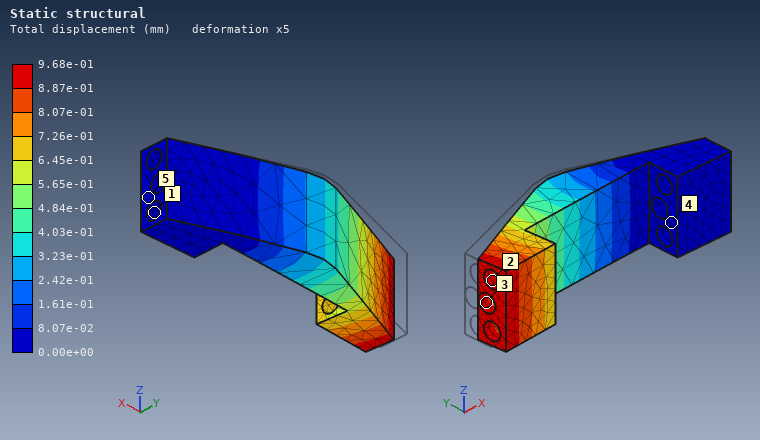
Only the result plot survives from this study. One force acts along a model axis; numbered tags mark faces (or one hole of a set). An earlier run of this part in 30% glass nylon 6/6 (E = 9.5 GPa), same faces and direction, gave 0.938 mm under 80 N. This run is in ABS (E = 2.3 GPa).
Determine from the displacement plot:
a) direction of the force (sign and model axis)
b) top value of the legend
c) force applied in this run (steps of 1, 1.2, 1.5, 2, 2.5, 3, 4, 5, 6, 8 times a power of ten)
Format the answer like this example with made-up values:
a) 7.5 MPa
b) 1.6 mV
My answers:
a) -Y
b) 9.68e-01 mm
c) 20 N
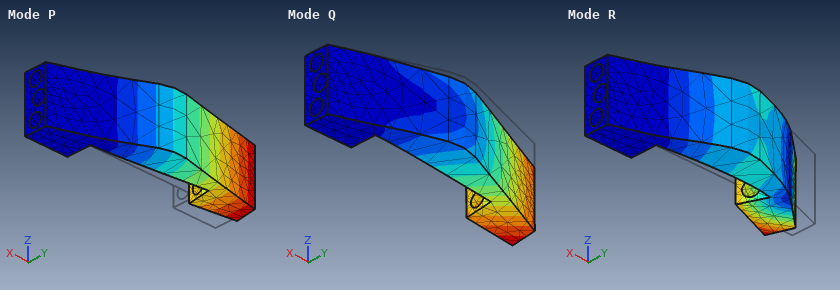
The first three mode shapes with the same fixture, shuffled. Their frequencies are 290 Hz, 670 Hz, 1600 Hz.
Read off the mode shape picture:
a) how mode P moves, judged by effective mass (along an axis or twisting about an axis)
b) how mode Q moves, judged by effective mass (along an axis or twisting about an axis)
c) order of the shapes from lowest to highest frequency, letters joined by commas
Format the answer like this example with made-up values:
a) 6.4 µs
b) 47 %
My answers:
a) along Y
b) along Z
c) P, Q, R
